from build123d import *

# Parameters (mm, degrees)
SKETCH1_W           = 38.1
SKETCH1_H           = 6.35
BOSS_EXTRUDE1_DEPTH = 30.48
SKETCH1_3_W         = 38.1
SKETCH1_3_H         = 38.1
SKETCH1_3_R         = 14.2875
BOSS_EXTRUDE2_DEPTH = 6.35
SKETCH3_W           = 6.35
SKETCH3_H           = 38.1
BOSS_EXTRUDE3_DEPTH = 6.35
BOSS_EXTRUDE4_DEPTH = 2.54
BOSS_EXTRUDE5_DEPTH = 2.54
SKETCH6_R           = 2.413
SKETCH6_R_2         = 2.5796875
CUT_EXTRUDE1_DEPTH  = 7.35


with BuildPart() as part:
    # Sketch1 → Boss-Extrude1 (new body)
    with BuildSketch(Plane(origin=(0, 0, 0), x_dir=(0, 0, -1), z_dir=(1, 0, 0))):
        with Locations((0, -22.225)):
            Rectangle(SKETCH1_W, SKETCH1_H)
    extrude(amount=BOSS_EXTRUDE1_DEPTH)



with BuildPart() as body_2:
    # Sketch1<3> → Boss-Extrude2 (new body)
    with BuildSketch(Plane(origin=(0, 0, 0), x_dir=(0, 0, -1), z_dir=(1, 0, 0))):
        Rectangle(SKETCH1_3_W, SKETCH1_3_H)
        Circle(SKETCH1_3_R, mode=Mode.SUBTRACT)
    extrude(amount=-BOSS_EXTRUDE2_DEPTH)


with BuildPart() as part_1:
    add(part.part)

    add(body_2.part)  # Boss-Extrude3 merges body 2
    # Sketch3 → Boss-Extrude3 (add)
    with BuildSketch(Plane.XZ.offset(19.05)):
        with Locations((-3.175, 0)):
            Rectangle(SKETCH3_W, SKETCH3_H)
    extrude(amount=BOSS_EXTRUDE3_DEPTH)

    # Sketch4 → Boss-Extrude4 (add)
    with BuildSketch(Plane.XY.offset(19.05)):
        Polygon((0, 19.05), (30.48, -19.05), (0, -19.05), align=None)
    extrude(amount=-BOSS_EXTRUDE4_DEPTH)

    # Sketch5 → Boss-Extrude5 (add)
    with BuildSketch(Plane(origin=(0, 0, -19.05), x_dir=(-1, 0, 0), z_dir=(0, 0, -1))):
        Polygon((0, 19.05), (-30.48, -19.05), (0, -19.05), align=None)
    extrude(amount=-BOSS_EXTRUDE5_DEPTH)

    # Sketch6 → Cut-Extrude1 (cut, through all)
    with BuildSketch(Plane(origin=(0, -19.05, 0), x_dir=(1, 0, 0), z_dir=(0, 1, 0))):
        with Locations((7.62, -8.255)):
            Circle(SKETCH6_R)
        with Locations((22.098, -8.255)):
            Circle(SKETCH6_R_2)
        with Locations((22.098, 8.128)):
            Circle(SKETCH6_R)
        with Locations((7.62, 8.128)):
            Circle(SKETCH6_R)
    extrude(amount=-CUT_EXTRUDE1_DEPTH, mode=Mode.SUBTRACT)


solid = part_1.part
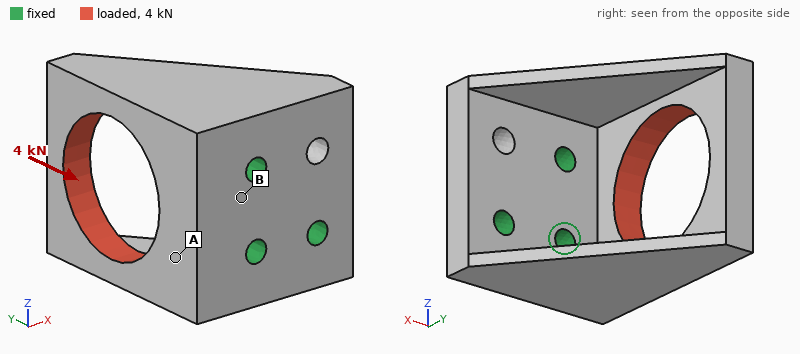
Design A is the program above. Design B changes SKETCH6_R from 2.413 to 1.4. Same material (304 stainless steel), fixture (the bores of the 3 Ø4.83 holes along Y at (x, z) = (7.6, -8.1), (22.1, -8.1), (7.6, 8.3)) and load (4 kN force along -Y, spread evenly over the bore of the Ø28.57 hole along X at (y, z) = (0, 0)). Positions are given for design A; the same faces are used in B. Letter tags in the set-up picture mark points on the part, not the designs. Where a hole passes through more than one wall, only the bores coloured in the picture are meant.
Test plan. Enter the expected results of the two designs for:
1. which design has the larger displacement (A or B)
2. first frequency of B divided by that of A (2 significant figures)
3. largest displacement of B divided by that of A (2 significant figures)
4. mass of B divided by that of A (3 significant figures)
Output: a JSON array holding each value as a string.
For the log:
["B", "0.93", "1.2", "1.01"]
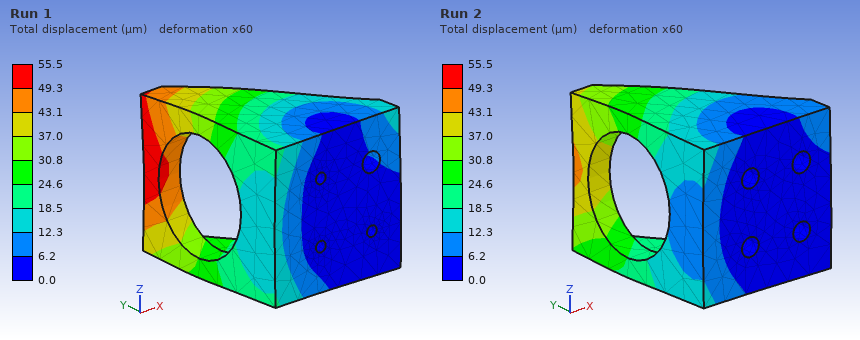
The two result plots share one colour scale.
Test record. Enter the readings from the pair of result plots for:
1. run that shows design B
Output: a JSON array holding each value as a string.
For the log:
["Run 1"]
